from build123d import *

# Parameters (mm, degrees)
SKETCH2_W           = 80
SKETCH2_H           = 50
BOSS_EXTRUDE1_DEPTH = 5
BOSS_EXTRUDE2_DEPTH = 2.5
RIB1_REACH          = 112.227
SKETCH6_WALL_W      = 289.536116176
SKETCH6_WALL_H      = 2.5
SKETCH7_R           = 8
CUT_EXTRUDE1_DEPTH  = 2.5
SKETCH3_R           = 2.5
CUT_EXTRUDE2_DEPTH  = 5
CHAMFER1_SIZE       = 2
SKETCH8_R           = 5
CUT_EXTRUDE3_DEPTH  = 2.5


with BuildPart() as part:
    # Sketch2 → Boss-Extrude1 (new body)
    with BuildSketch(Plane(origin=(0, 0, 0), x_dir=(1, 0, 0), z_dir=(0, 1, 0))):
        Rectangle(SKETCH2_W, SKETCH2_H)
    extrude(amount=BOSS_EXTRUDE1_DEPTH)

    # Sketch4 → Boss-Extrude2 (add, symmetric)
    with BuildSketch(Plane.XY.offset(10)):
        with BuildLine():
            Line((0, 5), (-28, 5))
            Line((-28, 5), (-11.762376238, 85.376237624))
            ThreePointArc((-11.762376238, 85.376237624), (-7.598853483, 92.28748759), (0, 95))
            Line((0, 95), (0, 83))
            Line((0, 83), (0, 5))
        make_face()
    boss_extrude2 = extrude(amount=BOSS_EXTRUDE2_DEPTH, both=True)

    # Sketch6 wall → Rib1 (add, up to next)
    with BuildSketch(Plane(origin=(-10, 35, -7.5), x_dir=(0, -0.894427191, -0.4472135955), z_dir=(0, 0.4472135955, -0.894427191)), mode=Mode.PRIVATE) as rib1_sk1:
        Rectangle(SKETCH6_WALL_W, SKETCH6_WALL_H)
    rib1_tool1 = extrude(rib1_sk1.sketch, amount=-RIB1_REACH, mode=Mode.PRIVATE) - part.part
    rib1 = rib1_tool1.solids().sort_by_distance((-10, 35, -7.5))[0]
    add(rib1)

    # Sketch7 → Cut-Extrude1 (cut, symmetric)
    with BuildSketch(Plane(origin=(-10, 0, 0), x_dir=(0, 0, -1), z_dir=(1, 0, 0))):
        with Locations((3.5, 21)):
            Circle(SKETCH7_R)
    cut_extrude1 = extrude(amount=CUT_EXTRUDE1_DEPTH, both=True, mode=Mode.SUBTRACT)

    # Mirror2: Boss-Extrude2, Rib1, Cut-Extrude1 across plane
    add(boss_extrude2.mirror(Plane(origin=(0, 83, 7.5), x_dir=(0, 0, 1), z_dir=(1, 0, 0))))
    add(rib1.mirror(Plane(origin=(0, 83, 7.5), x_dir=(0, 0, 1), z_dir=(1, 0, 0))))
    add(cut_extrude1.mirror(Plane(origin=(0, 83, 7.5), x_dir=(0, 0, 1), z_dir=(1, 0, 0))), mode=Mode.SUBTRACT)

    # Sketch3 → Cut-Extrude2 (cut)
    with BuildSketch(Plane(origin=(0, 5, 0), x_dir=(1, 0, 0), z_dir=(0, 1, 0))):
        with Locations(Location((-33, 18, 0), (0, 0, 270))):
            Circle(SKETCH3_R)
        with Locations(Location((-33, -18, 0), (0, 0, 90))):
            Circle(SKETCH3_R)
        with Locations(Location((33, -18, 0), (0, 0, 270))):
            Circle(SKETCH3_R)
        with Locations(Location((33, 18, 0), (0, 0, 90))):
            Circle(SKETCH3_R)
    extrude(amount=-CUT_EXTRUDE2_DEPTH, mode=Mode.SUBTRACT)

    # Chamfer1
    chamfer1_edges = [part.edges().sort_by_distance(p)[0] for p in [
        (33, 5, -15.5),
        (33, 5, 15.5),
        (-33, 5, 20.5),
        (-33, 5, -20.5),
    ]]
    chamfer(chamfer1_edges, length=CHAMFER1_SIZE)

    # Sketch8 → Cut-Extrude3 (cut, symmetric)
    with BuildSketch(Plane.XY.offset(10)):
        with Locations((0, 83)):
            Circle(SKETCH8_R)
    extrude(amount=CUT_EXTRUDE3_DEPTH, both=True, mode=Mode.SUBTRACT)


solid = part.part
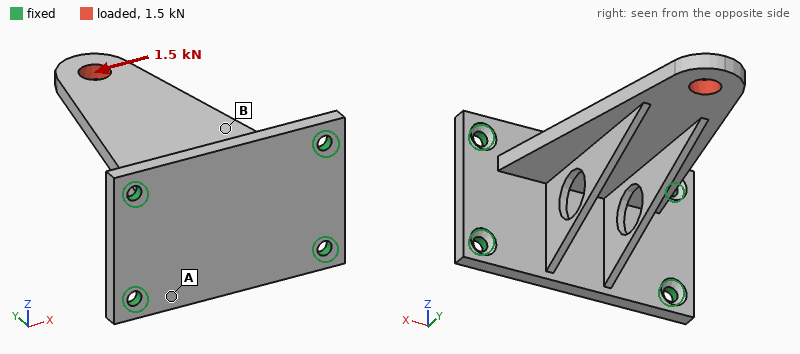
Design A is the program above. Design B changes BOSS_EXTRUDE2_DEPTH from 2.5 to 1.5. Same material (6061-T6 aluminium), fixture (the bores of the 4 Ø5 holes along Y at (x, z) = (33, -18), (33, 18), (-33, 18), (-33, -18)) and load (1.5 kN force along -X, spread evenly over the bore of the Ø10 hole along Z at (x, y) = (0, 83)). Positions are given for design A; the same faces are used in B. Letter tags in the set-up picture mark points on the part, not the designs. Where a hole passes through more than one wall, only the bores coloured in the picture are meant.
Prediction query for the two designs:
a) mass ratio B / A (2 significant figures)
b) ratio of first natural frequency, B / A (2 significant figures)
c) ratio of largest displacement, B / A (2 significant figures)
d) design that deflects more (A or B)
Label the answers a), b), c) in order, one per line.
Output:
a) 0.84
b) 1.1
c) 1.4
d) B
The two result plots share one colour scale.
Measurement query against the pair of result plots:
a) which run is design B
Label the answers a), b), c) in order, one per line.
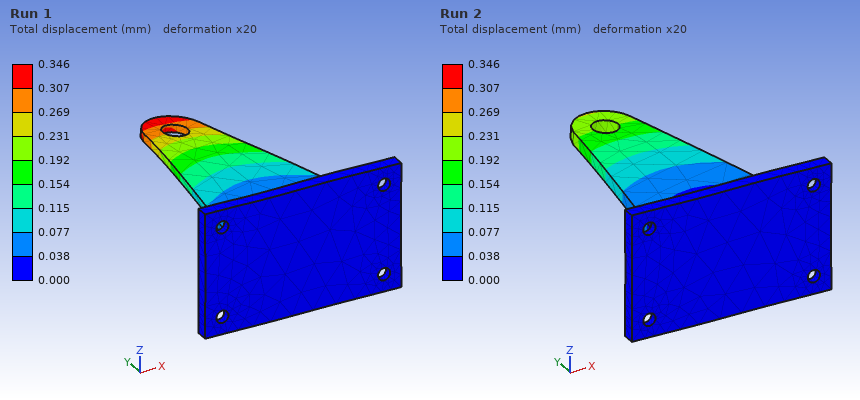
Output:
a) Run 1
